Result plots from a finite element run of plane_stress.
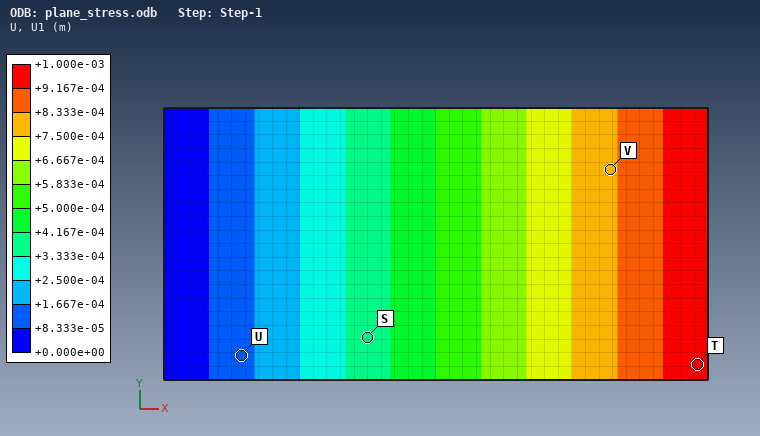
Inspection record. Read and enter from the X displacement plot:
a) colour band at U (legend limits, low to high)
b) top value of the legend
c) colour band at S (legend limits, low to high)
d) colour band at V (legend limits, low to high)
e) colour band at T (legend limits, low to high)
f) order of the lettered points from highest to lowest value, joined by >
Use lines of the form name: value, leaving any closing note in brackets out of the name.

colour band at U: +8.333e-05 to +1.667e-04 m
top value of the legend: +1.000e-03 m
colour band at S: +3.333e-04 to +4.167e-04 m
colour band at V: +7.500e-04 to +8.333e-04 m
colour band at T: +9.167e-04 to +1.000e-03 m
order of the lettered points from highest to lowest value, joined by >: T > V > S > U
